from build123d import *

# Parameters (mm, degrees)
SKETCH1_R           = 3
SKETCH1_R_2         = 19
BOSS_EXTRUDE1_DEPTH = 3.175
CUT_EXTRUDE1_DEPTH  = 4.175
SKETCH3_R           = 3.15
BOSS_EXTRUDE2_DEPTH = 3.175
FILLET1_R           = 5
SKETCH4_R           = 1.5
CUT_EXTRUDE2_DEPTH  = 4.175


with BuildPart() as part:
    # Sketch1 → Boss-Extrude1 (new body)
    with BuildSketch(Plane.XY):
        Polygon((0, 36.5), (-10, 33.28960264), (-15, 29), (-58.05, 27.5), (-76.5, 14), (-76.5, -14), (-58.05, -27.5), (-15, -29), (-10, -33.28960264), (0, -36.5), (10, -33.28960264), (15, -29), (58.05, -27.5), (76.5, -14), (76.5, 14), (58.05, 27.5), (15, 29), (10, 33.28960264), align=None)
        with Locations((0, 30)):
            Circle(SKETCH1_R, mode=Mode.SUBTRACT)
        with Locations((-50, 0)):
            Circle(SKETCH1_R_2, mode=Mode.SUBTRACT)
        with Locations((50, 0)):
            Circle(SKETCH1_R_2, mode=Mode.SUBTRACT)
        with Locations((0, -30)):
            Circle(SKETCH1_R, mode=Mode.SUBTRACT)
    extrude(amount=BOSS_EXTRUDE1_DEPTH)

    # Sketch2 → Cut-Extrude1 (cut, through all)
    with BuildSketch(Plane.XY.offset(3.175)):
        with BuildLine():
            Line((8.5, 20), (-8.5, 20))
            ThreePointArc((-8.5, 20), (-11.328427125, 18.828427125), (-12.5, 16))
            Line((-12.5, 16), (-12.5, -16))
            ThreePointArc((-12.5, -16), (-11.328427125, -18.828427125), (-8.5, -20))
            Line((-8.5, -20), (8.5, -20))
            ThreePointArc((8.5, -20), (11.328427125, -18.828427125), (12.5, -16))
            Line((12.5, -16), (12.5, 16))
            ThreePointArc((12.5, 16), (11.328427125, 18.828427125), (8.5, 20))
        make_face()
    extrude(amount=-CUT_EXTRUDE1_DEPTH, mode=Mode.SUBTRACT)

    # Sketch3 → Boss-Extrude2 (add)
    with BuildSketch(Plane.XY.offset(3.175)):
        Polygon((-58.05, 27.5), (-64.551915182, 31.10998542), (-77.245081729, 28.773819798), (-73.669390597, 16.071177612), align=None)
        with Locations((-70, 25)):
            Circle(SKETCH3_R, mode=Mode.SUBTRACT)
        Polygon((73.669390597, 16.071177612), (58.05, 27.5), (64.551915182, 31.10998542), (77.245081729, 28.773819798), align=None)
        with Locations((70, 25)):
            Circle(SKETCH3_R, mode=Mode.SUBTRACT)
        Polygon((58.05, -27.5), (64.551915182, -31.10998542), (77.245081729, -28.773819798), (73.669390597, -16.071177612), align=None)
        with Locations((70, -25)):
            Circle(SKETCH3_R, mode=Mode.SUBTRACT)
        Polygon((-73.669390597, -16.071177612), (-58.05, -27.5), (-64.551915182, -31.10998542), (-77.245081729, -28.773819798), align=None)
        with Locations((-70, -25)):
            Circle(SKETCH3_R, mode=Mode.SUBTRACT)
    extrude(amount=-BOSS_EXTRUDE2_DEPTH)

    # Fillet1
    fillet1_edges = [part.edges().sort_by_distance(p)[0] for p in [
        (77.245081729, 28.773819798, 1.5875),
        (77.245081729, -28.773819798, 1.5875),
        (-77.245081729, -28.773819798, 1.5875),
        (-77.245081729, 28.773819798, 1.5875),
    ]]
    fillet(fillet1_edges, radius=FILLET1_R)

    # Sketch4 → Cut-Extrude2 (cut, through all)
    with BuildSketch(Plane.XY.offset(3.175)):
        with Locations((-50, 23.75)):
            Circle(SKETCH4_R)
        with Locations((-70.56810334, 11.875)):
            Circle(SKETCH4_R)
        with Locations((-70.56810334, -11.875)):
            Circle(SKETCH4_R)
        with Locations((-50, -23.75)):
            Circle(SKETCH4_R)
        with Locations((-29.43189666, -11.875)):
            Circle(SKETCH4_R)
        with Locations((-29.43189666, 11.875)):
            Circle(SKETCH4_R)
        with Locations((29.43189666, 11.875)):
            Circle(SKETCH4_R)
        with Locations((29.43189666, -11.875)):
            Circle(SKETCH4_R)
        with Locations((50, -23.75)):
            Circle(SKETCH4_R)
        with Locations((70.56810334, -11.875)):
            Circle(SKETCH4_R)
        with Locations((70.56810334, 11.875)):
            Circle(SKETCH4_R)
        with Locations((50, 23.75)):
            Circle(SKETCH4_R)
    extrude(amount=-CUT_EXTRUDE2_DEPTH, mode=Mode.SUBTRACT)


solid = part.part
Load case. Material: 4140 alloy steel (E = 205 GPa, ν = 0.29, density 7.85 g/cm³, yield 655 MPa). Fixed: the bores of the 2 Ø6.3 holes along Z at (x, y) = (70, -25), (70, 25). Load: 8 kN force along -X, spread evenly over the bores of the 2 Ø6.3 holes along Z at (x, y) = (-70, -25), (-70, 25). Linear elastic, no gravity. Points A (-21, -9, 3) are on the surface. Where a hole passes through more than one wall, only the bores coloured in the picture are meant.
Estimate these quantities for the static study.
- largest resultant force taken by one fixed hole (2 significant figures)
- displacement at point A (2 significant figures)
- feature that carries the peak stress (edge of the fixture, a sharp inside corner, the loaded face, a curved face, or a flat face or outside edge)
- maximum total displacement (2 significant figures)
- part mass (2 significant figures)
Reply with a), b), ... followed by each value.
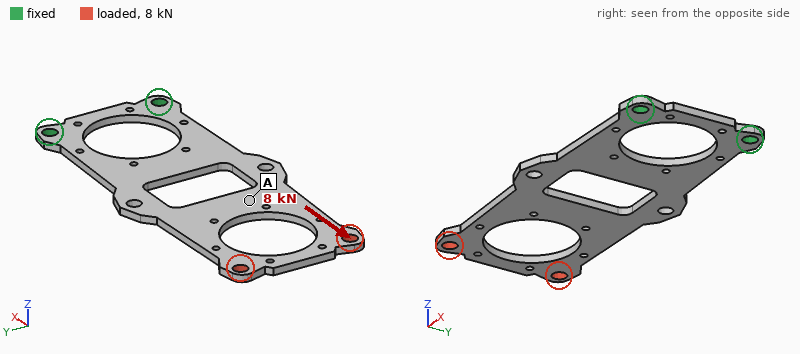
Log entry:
a) 4.0 kN
b) 63 µm
c) a curved face
d) 96 µm
e) 140 g
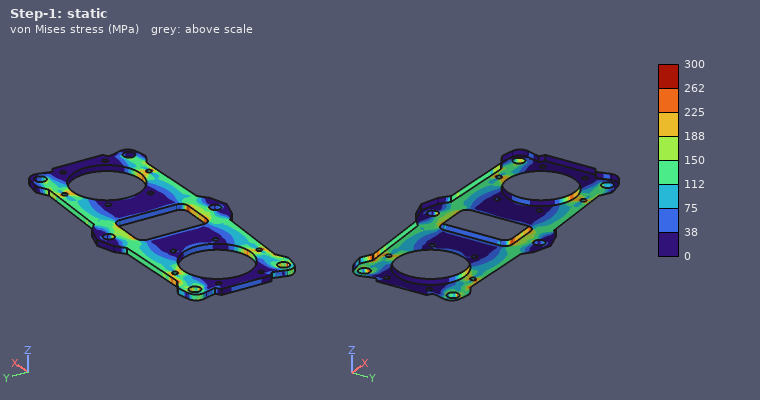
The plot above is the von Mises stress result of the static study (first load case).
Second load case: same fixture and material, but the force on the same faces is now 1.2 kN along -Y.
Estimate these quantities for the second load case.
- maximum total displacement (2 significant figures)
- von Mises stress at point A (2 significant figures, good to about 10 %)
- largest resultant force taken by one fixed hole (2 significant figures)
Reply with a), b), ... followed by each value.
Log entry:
a) 0.30 mm
b) 34 MPa
c) 3.2 kN
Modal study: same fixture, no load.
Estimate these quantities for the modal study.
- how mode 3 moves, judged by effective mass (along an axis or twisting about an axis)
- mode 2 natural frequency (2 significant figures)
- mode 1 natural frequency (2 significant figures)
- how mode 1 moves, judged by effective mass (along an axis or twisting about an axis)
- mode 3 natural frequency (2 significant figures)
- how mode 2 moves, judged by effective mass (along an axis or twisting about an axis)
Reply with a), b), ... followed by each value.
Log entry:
a) along Z
b) 530 Hz
c) 100 Hz
d) along Z
e) 620 Hz
f) twisting about X
